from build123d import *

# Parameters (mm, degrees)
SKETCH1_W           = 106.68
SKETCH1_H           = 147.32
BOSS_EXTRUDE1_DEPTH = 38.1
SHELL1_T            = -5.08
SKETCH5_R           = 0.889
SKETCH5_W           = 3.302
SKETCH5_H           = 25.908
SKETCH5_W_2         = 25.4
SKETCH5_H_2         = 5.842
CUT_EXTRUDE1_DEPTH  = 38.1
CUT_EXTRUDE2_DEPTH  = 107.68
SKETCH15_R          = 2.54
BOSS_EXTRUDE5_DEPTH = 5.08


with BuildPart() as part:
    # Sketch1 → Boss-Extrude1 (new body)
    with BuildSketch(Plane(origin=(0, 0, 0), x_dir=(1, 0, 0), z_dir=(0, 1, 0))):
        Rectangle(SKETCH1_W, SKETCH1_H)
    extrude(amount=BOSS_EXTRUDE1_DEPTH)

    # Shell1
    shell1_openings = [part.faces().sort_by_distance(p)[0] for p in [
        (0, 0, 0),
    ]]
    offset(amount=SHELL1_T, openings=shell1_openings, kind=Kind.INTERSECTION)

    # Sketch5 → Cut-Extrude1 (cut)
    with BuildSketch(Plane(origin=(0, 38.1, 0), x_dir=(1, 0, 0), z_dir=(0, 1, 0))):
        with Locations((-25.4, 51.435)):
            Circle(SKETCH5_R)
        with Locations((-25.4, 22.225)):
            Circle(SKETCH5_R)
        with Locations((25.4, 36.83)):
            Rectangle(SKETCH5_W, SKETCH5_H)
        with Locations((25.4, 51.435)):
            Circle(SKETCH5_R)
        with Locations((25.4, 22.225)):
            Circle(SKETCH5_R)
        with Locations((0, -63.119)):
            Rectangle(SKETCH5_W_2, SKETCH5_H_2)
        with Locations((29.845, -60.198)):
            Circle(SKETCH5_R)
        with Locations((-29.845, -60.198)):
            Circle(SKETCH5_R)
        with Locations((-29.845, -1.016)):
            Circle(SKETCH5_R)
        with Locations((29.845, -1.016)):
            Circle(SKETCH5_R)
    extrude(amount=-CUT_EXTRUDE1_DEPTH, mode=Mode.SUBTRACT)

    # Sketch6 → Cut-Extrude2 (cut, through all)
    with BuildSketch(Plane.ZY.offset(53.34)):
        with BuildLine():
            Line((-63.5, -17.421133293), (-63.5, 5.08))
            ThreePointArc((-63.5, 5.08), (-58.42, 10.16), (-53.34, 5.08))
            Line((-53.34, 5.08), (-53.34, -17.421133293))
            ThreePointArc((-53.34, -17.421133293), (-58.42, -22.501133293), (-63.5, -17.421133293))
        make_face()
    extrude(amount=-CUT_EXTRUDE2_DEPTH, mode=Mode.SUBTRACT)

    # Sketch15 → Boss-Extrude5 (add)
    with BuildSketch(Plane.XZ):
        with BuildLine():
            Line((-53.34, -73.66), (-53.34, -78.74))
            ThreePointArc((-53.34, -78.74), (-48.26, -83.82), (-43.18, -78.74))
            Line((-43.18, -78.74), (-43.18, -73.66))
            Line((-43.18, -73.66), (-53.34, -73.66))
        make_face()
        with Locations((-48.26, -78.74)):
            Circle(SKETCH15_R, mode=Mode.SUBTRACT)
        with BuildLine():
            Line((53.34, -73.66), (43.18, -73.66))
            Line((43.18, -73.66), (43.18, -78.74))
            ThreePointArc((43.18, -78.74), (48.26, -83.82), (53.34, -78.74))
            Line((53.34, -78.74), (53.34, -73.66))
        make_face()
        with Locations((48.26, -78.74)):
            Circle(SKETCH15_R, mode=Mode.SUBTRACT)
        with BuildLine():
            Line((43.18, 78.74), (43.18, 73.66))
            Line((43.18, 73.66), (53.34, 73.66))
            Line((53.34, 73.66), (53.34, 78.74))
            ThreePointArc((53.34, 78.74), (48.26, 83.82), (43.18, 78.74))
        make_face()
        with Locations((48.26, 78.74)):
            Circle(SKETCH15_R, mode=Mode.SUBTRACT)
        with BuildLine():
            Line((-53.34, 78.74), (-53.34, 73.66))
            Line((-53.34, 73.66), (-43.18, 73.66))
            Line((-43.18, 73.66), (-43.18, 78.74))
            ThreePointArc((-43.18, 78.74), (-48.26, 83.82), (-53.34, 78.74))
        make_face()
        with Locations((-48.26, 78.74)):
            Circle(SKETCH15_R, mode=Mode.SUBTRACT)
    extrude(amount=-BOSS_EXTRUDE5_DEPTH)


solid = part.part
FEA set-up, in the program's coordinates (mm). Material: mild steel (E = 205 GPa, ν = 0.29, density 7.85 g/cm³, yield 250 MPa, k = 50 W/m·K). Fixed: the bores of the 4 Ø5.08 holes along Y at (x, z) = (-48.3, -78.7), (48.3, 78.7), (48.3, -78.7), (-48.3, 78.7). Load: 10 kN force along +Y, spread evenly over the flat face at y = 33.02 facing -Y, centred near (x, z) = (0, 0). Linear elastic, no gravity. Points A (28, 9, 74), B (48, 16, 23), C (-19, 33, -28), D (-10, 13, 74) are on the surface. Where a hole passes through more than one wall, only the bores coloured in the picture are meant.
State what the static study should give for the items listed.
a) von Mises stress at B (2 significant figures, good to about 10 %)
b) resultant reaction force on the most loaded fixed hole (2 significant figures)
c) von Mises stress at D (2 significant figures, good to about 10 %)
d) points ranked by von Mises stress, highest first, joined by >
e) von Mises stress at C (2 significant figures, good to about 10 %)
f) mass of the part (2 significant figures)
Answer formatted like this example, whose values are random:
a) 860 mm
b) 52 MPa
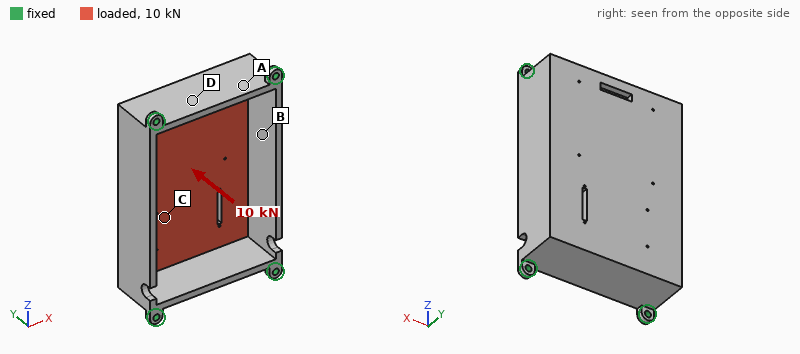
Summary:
a) 39 MPa
b) 3.1 kN
c) 21 MPa
d) C > B > D > A
e) 55 MPa
f) 1.3 kg
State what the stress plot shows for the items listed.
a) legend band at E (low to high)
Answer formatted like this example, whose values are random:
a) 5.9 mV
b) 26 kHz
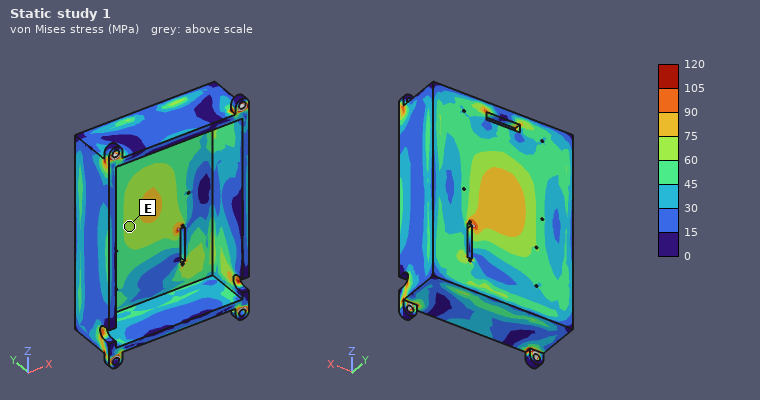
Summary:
a) 60 to 75 MPa
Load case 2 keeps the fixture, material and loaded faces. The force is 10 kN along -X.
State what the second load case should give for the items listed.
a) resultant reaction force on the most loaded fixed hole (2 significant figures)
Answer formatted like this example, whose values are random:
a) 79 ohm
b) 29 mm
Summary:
a) 3.1 kN
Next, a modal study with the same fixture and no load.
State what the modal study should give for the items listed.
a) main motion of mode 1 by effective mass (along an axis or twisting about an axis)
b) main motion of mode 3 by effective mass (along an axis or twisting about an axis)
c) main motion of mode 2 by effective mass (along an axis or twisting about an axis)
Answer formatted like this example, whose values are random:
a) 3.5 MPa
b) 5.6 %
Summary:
a) along Y
b) along Y
c) along X
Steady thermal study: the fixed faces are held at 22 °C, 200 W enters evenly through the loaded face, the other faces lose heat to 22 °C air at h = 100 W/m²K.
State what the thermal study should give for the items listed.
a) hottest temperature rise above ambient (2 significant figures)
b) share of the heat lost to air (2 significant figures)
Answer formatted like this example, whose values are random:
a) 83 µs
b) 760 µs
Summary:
a) 75 K
b) 90 %
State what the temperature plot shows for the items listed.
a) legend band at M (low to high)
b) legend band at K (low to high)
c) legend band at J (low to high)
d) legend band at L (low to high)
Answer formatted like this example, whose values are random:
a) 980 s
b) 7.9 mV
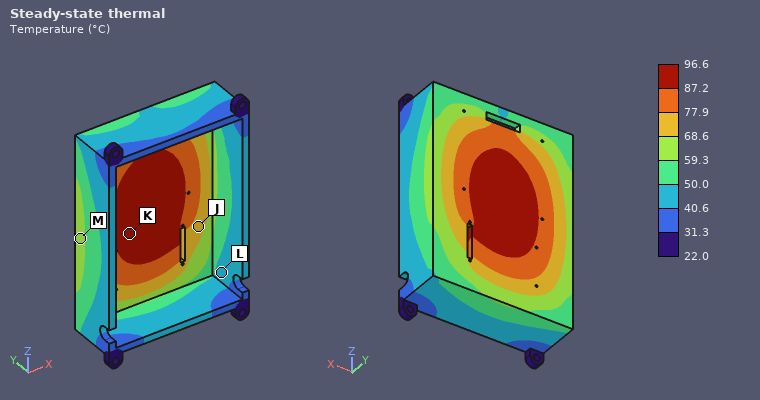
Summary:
a) 59.3 to 68.6 °C
b) 87.2 to 96.6 °C
c) 68.6 to 77.9 °C
d) 40.6 to 50.0 °C
